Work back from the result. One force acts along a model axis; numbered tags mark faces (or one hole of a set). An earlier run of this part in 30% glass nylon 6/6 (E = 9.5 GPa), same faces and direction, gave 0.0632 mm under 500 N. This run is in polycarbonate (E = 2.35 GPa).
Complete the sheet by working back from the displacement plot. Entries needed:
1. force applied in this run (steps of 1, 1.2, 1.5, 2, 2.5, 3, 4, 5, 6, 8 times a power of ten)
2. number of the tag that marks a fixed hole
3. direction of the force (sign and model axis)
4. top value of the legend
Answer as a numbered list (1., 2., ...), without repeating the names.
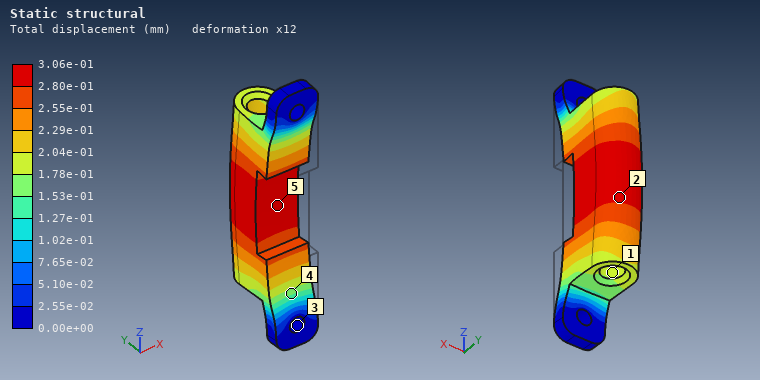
1. 600 N
2. 3
3. +Y
4. 3.06e-01 mm
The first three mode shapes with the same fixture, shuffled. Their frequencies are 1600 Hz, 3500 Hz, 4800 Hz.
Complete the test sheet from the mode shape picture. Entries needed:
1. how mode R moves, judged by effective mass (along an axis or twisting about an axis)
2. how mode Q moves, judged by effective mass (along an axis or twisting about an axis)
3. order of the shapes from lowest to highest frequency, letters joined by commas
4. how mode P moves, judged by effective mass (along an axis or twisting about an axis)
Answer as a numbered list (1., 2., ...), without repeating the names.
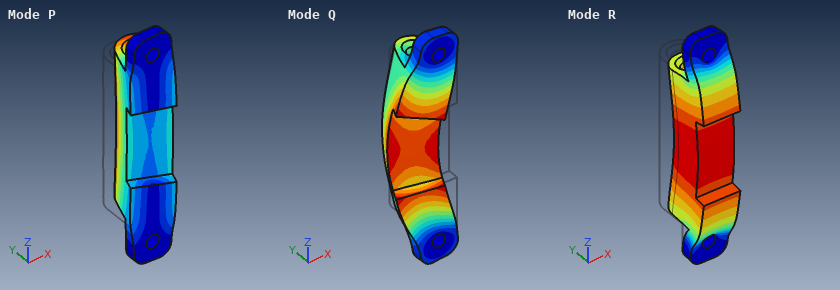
1. along Y
2. along X
3. P, R, Q
4. along X
